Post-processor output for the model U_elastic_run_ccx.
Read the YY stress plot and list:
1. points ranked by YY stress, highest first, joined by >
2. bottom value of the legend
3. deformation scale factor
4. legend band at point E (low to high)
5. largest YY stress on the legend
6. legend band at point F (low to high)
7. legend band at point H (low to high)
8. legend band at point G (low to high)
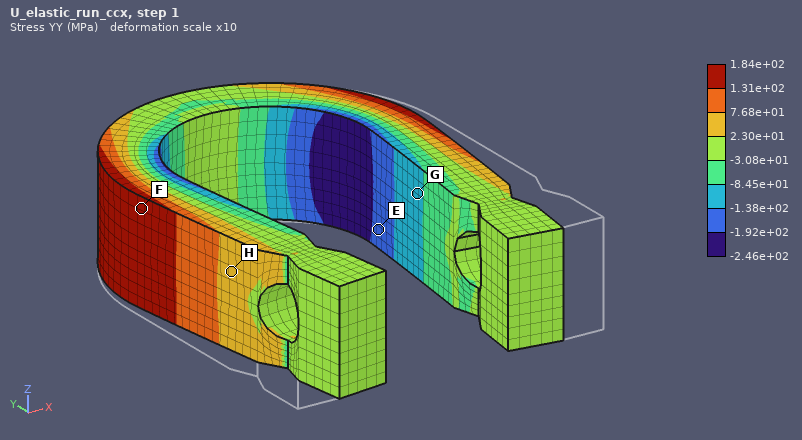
F > H > G > E
-2.46e+02 MPa
10
-1.92e+02 to -1.38e+02 MPa
1.84e+02 MPa
1.31e+02 to 1.84e+02 MPa
2.30e+01 to 7.68e+01 MPa
-1.38e+02 to -8.45e+01 MPa
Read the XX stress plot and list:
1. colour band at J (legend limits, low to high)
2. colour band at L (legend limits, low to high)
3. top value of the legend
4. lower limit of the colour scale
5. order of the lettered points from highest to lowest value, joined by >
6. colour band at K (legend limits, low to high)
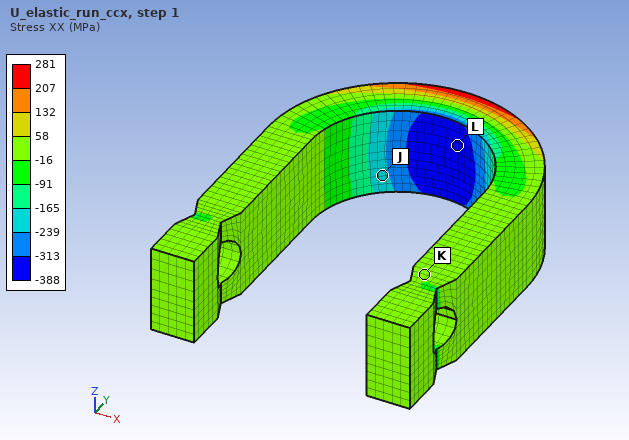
-239 to -165 MPa
-388 to -313 MPa
281 MPa
-388 MPa
K > J > L
-16 to 58 MPa
